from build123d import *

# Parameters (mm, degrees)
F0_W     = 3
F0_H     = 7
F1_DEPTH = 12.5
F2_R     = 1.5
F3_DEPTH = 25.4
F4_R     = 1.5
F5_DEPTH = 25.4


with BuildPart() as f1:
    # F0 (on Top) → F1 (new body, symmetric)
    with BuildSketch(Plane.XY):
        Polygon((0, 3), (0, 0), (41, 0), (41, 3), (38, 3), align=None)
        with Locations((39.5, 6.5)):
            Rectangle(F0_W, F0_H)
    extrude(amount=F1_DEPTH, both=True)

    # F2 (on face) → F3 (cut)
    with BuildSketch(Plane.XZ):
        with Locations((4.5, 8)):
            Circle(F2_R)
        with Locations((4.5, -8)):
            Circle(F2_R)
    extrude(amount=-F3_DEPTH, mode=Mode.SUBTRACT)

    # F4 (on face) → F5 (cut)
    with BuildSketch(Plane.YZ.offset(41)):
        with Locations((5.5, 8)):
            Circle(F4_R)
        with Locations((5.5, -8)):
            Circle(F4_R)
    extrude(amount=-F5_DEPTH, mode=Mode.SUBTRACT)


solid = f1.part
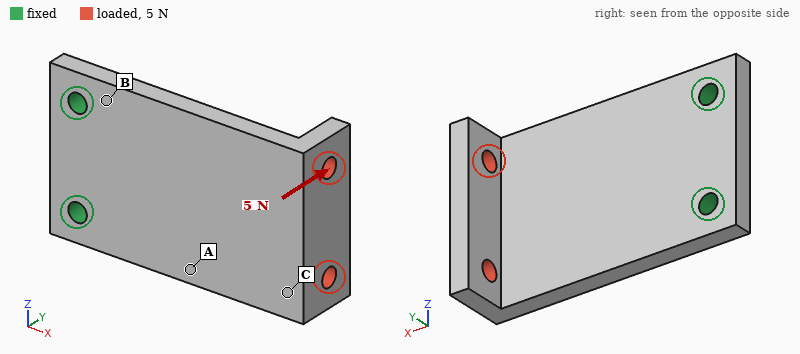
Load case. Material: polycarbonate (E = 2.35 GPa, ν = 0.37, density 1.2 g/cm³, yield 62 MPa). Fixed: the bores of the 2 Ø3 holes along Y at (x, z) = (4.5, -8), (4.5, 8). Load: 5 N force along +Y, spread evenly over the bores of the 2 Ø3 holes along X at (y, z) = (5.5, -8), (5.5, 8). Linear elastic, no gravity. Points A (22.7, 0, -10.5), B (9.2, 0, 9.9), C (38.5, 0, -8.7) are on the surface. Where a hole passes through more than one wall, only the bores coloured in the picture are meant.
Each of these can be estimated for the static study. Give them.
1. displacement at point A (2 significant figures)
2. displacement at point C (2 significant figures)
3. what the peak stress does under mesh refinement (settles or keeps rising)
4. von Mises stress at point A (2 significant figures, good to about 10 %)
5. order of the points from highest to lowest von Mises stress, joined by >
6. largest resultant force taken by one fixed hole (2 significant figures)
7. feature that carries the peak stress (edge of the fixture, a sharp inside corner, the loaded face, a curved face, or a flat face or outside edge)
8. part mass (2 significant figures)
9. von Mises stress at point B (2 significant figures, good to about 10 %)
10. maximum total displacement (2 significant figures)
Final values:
0.17 mm
0.50 mm
keeps rising
2.3 MPa
B > A > C
2.5 N
edge of the fixture
4.2 g
4.2 MPa
0.59 mm
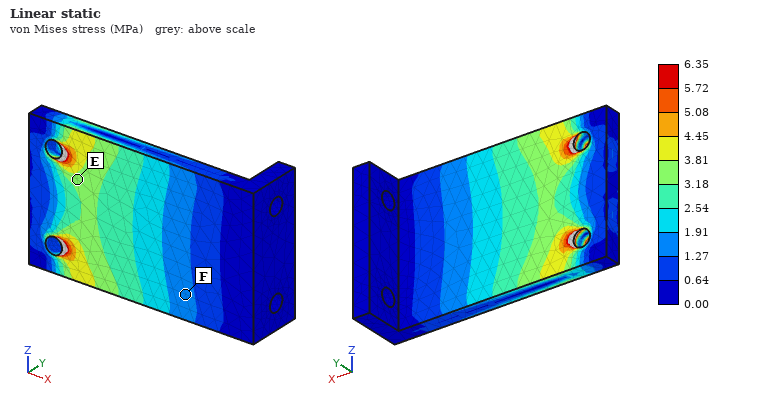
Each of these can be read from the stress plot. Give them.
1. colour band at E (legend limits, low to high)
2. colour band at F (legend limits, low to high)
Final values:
3.18 to 3.81 MPa
1.27 to 1.91 MPa
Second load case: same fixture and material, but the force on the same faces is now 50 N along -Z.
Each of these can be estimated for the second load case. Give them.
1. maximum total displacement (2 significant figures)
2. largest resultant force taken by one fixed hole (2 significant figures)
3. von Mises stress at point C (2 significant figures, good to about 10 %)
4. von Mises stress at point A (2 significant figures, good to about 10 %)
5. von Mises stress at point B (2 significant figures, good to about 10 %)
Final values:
0.51 mm
100 N
2.5 MPa
4.3 MPa
7.3 MPa
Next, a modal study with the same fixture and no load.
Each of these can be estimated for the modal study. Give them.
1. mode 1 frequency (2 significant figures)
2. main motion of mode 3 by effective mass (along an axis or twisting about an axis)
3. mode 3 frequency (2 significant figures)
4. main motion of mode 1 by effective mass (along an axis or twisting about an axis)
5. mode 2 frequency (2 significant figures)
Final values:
400 Hz
along Y
2500 Hz
along Y
1300 Hz
